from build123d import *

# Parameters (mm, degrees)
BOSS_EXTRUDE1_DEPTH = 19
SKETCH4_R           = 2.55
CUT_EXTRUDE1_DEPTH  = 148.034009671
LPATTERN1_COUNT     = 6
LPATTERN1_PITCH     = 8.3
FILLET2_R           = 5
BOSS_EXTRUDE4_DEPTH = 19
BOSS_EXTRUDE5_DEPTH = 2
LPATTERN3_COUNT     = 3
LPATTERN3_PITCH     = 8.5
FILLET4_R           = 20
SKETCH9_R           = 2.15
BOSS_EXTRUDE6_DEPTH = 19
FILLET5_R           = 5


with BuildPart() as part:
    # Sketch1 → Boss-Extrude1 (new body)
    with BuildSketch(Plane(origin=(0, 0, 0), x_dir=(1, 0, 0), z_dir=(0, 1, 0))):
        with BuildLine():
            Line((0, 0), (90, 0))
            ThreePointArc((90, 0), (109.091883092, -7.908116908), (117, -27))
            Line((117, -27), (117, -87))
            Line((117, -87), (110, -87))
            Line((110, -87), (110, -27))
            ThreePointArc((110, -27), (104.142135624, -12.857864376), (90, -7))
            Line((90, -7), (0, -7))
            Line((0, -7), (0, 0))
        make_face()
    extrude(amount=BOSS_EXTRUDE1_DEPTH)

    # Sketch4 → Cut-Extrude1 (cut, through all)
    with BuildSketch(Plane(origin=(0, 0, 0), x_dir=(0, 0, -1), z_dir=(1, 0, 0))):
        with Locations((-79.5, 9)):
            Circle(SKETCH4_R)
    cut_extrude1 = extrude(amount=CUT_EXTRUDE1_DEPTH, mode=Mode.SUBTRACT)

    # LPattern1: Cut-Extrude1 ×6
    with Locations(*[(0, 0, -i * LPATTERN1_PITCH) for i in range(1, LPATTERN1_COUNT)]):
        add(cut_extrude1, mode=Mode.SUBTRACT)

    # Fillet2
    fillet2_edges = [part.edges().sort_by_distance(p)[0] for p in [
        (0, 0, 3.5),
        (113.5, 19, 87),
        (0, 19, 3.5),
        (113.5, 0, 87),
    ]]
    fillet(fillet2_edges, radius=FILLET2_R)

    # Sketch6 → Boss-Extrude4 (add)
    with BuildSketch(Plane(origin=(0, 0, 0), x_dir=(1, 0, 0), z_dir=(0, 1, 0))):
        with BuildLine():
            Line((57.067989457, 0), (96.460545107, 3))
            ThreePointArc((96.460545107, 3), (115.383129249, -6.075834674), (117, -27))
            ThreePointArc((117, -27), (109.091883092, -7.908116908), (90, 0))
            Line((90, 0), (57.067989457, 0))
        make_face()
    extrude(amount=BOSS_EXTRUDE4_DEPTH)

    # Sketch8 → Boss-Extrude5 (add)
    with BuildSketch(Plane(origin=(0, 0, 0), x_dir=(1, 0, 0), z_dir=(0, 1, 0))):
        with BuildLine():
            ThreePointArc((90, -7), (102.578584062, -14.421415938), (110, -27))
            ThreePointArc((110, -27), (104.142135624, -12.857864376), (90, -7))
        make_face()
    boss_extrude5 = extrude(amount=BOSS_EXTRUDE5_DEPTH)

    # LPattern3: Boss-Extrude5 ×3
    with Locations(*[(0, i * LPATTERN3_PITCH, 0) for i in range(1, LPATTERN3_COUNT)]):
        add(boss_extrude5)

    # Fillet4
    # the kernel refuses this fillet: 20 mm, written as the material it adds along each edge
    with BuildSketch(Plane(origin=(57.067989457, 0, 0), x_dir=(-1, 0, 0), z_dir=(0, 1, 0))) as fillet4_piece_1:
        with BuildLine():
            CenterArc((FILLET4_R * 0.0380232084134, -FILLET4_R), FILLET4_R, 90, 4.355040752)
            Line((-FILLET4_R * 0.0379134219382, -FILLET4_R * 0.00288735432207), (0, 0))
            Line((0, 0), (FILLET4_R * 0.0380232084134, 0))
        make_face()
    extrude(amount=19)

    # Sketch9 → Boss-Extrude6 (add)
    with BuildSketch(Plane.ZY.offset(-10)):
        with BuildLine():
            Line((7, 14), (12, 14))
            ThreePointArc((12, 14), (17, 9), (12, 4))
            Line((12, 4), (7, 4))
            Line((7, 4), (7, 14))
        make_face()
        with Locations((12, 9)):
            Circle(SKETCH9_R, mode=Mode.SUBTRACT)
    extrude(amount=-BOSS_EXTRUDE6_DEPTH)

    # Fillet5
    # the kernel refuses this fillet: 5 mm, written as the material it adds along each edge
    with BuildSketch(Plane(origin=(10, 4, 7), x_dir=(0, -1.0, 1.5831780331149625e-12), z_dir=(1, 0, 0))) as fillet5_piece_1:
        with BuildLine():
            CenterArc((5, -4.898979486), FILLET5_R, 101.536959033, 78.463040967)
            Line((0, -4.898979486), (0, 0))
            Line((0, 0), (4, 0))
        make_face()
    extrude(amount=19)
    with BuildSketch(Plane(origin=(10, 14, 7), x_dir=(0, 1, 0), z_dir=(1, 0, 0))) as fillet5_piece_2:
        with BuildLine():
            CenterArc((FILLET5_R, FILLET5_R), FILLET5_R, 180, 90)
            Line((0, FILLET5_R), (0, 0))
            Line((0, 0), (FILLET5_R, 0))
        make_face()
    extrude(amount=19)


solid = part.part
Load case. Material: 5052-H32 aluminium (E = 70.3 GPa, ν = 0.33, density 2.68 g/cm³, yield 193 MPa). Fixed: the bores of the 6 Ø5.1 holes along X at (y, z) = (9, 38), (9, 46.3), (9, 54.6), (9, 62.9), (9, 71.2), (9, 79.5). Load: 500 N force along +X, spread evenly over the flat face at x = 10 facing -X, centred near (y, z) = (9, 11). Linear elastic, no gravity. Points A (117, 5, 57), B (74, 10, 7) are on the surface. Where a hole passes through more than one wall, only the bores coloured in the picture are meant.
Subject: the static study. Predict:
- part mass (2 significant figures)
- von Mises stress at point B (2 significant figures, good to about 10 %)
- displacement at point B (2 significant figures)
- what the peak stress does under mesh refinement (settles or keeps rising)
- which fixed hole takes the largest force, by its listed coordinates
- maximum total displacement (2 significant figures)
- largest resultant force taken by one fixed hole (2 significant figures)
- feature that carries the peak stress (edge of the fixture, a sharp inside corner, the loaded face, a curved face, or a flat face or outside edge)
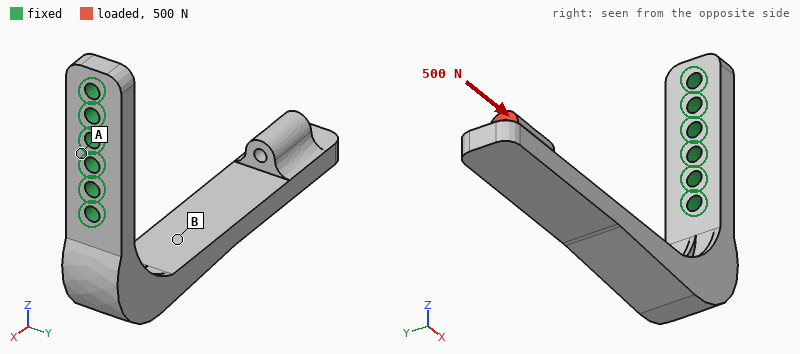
81 g
22 MPa
0.17 mm
keeps rising
(9, 38)
0.21 mm
820 N
edge of the fixture
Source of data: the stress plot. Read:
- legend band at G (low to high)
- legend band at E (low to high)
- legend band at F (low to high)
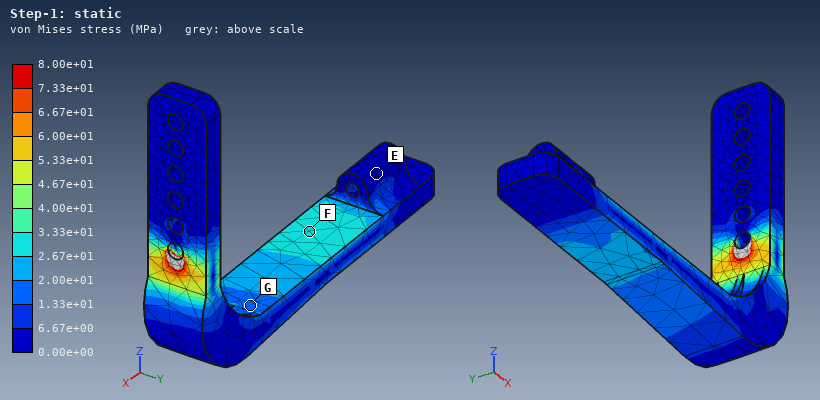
1.33e+01 to 2.00e+01 MPa
0.00e+00 to 6.67e+00 MPa
2.67e+01 to 3.33e+01 MPa
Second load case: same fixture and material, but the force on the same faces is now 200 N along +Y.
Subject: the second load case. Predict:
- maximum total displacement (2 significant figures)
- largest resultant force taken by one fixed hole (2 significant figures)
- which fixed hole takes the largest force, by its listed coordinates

1.1 mm
420 N
(9, 38)
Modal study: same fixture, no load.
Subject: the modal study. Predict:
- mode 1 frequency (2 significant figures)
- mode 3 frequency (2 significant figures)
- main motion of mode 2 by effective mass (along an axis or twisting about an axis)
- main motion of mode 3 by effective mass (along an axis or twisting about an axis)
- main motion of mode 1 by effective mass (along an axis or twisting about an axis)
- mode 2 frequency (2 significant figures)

410 Hz
1600 Hz
along Y
along X
along Z
530 Hz
